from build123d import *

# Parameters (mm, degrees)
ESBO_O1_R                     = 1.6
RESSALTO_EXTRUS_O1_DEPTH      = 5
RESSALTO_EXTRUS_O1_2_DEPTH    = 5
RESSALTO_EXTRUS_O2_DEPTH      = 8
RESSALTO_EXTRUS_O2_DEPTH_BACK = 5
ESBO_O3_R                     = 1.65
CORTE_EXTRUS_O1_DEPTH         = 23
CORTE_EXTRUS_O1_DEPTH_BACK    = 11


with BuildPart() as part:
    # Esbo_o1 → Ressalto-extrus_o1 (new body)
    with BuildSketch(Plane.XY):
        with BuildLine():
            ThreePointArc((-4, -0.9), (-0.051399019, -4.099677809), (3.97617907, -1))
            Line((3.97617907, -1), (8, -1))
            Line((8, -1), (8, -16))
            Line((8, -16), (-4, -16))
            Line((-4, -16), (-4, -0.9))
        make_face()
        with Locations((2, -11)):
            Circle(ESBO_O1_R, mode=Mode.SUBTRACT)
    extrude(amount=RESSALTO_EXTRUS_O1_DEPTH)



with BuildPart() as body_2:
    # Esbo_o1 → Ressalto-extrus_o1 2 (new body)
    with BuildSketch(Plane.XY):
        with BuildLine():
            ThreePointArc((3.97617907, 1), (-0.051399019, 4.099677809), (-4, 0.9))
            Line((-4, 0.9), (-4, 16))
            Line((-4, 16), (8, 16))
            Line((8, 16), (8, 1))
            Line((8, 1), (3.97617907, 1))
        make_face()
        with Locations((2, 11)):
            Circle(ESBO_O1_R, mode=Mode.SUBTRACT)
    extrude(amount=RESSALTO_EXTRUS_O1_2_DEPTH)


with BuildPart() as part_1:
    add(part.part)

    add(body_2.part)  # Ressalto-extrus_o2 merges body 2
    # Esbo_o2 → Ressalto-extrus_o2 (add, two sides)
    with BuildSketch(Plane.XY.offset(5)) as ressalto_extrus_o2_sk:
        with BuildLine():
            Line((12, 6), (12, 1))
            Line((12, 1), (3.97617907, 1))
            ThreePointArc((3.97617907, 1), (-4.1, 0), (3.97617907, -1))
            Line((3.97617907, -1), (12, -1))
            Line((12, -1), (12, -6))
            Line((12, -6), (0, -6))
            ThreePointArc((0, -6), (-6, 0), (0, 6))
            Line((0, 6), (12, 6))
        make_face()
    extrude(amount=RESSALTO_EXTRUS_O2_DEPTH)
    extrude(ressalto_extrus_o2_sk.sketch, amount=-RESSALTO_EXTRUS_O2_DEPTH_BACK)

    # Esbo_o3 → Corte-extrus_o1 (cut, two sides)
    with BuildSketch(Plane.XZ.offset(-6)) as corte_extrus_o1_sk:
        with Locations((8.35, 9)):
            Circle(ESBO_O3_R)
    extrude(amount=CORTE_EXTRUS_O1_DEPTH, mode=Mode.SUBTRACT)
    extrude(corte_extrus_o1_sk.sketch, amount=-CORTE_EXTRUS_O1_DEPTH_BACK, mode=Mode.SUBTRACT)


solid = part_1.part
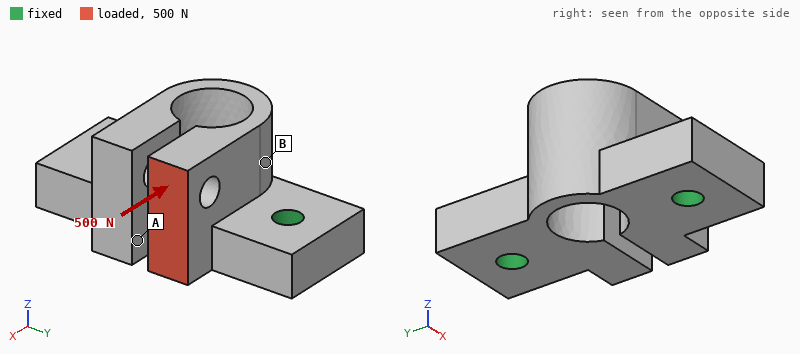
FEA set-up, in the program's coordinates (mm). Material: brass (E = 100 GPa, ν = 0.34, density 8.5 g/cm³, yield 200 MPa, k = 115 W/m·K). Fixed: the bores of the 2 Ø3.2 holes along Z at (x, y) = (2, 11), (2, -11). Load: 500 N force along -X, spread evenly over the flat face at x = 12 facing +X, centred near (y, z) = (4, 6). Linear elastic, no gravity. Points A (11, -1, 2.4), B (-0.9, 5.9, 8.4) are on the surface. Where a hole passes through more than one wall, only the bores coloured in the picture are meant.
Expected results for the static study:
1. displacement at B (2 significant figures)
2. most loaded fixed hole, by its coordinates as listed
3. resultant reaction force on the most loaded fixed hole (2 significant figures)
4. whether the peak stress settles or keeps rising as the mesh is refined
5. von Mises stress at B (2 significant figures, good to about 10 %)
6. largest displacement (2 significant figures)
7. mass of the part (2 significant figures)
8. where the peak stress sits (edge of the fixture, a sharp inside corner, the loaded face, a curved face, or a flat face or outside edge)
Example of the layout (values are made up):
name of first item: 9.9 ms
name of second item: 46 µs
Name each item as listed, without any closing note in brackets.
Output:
displacement at B: 8.1 µm
most loaded fixed hole, by its coordinates as listed: (2, 11)
resultant reaction force on the most loaded fixed hole: 460 N
whether the peak stress settles or keeps rising as the mesh is refined: keeps rising
von Mises stress at B: 18 MPa
largest displacement: 18 µm
mass of the part: 24 g
where the peak stress sits: edge of the fixture
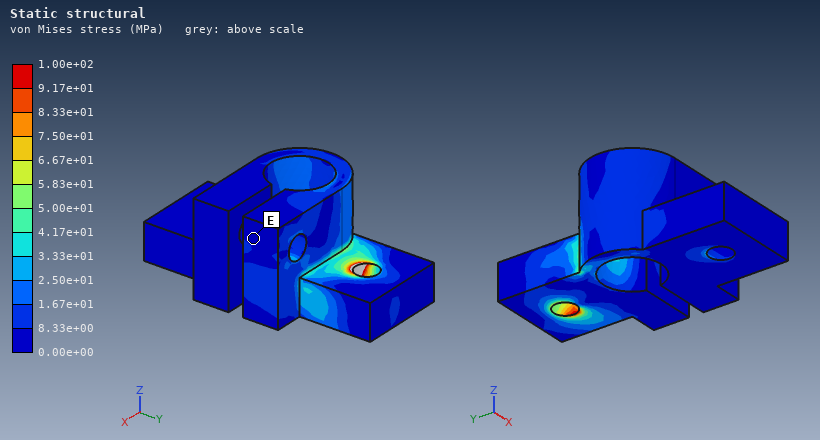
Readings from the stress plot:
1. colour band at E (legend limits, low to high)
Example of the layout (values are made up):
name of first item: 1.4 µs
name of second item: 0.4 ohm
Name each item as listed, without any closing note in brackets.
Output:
colour band at E: 0.00e+00 to 8.33e+00 MPa
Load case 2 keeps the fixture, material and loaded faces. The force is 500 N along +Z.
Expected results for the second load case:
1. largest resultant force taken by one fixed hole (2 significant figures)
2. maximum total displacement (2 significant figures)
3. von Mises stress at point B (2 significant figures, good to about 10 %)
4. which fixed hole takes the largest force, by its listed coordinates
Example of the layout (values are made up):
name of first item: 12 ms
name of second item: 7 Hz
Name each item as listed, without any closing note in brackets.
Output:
largest resultant force taken by one fixed hole: 530 N
maximum total displacement: 44 µm
von Mises stress at point B: 34 MPa
which fixed hole takes the largest force, by its listed coordinates: (2, 11)
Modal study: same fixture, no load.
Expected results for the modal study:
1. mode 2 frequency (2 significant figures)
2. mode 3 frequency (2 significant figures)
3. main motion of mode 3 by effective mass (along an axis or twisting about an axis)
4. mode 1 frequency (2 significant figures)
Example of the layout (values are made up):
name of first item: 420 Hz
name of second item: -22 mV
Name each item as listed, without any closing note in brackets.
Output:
mode 2 frequency: 10 kHz
mode 3 frequency: 12 kHz
main motion of mode 3 by effective mass: along X
mode 1 frequency: 10 kHz
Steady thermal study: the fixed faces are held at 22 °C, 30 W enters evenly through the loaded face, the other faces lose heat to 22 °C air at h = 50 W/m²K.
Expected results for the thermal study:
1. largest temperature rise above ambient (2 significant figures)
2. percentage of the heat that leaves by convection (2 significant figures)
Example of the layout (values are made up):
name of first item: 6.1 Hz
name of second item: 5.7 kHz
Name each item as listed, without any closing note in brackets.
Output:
largest temperature rise above ambient: 74 K
percentage of the heat that leaves by convection: 4.8 %
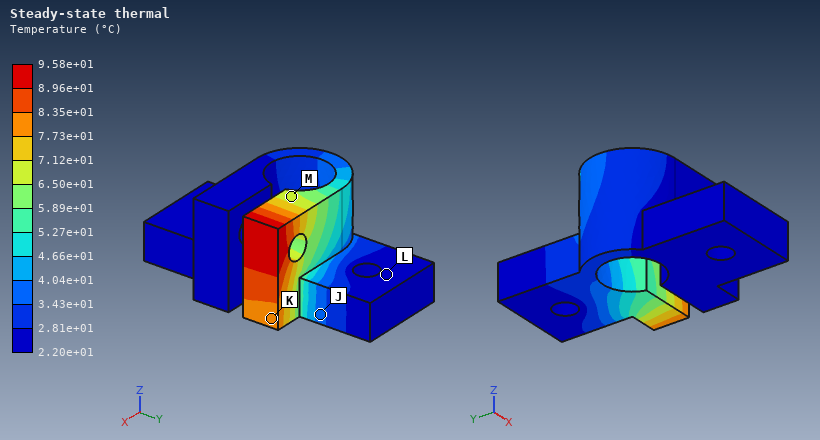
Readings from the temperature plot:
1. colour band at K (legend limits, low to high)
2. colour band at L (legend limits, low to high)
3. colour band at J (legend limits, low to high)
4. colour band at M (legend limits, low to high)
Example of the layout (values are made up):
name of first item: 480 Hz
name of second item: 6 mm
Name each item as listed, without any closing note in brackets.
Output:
colour band at K: 7.73e+01 to 8.35e+01 °C
colour band at L: 2.20e+01 to 2.81e+01 °C
colour band at J: 3.43e+01 to 4.04e+01 °C
colour band at M: 6.50e+01 to 7.12e+01 °C
